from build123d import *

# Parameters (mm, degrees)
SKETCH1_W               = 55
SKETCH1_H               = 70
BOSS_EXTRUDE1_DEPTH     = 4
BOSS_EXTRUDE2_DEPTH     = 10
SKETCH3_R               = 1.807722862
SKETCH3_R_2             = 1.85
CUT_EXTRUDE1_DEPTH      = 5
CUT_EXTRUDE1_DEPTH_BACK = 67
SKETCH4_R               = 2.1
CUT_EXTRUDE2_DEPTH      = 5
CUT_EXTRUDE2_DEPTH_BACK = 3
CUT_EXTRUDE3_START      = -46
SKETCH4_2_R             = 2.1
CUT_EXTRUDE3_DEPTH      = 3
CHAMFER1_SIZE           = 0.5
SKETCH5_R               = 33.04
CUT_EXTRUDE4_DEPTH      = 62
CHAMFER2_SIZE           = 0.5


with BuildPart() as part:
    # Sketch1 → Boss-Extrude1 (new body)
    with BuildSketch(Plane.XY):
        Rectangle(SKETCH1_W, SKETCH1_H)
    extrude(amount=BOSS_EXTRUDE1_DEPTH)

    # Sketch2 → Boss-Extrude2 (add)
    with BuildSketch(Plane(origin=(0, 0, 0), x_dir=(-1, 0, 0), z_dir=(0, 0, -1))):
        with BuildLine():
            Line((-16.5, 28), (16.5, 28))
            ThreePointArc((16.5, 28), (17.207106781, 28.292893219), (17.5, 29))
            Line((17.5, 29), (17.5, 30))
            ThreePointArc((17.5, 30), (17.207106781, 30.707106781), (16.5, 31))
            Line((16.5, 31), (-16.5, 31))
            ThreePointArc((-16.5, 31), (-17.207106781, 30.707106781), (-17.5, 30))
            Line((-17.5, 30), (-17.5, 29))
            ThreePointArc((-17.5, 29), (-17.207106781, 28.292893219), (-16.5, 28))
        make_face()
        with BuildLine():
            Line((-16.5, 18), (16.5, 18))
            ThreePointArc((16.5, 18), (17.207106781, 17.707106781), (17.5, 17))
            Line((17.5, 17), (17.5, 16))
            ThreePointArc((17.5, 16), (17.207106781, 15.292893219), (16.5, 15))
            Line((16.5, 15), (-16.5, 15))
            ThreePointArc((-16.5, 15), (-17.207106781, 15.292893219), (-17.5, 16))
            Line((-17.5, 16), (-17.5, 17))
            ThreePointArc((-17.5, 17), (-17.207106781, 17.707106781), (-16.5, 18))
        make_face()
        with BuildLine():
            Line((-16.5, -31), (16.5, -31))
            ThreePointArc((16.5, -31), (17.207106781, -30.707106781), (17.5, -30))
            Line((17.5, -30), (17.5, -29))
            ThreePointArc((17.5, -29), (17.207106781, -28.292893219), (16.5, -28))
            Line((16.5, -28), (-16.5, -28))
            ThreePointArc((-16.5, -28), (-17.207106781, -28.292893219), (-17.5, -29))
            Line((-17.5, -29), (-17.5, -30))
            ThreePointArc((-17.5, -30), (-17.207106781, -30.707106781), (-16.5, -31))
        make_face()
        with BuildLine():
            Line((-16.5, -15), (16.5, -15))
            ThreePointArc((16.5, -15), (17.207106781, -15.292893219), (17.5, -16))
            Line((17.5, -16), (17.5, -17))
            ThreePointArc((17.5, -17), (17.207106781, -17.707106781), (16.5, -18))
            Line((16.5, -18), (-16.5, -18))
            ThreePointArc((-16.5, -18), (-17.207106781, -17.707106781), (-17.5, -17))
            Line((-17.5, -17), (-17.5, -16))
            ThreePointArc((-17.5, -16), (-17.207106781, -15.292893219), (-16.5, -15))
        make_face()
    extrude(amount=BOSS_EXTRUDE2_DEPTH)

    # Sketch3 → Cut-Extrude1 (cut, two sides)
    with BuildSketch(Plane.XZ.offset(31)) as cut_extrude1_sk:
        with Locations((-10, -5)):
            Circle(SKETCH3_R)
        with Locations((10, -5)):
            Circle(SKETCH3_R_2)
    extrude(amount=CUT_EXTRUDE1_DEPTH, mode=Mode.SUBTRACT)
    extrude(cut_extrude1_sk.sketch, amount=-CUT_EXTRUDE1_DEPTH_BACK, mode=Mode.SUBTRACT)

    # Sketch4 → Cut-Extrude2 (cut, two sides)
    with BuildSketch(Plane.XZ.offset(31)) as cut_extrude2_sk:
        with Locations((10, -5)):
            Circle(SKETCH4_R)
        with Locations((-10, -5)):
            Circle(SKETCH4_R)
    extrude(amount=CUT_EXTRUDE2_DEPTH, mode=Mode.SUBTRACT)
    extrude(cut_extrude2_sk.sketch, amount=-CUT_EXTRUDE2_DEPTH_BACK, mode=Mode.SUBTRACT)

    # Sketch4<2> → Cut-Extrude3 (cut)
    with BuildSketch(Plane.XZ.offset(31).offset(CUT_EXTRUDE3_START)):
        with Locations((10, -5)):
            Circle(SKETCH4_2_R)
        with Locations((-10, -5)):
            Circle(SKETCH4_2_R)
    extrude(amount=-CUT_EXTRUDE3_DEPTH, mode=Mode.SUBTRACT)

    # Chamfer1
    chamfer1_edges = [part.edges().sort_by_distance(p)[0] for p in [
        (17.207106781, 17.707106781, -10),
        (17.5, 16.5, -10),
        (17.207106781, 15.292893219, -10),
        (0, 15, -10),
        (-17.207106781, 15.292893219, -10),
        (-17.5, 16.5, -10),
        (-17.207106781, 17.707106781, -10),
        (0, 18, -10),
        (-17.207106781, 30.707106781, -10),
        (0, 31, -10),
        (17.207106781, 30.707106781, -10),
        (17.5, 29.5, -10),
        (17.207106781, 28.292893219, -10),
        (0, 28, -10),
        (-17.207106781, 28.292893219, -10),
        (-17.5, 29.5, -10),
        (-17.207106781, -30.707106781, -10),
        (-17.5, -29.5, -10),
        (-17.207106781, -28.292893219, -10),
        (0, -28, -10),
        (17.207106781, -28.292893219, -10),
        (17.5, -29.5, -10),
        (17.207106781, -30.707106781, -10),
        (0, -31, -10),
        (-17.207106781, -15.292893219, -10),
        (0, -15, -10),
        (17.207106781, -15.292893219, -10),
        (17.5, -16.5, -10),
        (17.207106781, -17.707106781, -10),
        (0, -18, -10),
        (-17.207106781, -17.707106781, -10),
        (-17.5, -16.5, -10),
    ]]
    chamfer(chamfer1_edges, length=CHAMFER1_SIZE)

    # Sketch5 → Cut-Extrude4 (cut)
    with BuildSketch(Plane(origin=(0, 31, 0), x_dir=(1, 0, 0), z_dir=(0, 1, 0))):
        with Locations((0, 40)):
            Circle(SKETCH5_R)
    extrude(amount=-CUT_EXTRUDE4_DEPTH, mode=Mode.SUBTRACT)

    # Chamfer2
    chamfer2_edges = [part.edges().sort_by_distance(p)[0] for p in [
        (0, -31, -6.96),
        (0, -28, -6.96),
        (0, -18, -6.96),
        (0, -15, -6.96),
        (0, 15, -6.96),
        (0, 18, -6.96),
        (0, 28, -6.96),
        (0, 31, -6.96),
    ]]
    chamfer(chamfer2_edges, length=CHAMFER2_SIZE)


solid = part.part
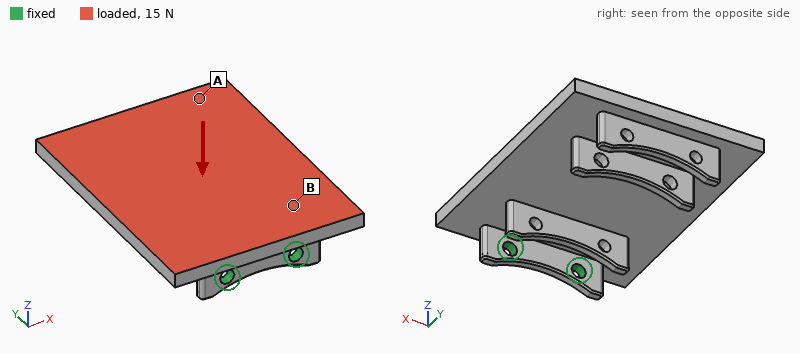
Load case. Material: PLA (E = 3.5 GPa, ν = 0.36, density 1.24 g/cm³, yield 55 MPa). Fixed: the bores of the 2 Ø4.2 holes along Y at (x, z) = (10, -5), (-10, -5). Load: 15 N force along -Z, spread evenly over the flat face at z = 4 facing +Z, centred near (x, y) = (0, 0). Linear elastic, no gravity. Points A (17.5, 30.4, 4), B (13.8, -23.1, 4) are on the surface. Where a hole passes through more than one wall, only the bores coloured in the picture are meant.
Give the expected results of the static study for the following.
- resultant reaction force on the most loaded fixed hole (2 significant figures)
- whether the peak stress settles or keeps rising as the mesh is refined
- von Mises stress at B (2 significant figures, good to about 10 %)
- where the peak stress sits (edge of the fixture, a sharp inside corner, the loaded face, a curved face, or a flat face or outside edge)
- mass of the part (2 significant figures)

8.7 N
keeps rising
2.2 MPa
edge of the fixture
23 g
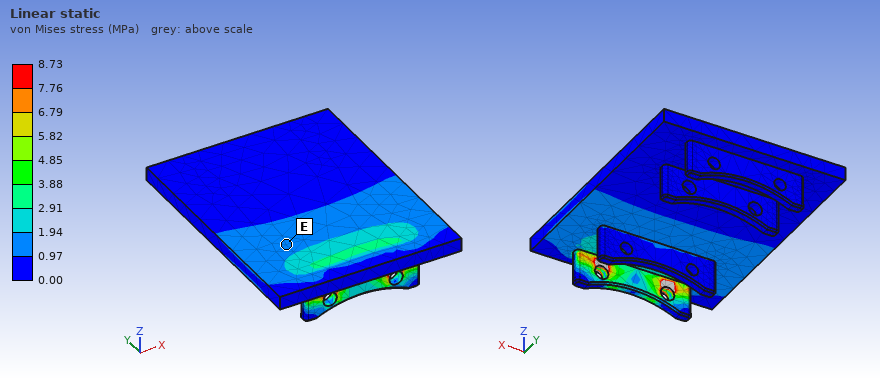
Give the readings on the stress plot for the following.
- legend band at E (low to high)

0.97 to 1.94 MPa
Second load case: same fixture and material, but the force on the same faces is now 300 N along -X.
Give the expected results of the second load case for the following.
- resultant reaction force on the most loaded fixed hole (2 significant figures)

430 N
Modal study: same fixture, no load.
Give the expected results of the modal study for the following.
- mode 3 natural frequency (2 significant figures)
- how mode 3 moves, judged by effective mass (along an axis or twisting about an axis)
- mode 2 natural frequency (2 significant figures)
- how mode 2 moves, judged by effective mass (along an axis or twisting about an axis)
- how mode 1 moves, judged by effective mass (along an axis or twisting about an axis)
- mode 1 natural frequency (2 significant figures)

740 Hz
along X
530 Hz
along X
along Z
160 Hz
